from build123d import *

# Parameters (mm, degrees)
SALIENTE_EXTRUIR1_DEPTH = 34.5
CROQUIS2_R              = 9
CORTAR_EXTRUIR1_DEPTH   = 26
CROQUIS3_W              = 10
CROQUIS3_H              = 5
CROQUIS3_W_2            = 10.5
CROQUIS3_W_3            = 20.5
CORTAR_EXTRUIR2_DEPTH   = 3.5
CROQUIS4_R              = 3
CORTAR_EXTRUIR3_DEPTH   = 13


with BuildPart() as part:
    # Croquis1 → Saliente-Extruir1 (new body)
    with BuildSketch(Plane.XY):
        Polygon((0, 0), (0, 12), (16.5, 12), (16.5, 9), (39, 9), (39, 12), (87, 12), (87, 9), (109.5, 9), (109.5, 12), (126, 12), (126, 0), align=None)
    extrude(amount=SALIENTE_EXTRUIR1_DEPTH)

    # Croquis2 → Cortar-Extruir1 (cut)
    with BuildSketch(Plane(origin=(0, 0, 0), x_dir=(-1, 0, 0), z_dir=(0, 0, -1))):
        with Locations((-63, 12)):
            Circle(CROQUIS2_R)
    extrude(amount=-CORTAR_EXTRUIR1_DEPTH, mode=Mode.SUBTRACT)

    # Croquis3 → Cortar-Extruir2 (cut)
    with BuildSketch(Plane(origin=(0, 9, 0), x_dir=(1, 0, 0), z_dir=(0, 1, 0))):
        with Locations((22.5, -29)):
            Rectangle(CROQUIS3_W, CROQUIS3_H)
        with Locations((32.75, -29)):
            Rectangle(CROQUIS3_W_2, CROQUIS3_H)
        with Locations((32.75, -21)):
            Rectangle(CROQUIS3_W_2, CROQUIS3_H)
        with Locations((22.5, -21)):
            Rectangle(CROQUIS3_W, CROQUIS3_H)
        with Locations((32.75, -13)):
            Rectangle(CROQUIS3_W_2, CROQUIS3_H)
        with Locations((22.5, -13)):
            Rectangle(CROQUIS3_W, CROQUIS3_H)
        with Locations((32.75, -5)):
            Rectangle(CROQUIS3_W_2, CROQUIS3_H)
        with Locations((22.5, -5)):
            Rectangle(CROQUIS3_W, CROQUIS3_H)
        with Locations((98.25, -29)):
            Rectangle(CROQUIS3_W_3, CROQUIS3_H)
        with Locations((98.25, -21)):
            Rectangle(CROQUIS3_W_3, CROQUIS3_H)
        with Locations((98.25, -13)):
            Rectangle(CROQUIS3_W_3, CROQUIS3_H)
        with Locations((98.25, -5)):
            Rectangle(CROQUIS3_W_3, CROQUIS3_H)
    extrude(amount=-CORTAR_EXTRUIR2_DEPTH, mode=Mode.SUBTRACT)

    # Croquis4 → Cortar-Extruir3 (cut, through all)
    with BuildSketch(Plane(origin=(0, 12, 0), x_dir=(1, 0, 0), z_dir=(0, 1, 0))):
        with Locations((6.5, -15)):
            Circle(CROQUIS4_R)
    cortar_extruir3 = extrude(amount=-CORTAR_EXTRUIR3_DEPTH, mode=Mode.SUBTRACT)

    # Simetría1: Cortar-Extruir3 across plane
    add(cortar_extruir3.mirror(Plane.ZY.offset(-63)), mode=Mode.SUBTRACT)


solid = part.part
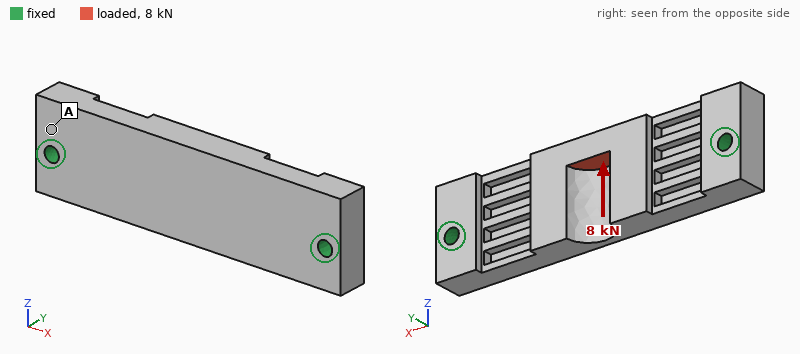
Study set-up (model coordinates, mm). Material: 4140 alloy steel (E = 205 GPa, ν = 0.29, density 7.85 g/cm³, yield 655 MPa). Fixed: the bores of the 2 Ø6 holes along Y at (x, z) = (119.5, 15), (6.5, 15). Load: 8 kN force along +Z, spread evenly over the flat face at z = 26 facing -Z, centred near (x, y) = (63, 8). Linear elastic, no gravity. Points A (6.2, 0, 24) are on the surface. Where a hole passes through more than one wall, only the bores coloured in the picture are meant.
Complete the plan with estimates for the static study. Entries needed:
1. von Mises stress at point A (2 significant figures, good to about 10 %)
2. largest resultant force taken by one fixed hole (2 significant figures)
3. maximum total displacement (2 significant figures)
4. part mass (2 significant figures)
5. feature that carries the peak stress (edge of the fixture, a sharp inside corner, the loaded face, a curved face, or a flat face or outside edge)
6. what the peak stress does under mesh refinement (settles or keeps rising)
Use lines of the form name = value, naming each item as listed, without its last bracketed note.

von Mises stress at point A = 43 MPa
largest resultant force taken by one fixed hole = 5.0 kN
maximum total displacement = 84 µm
part mass = 320 g
feature that carries the peak stress = edge of the fixture
what the peak stress does under mesh refinement = keeps rising
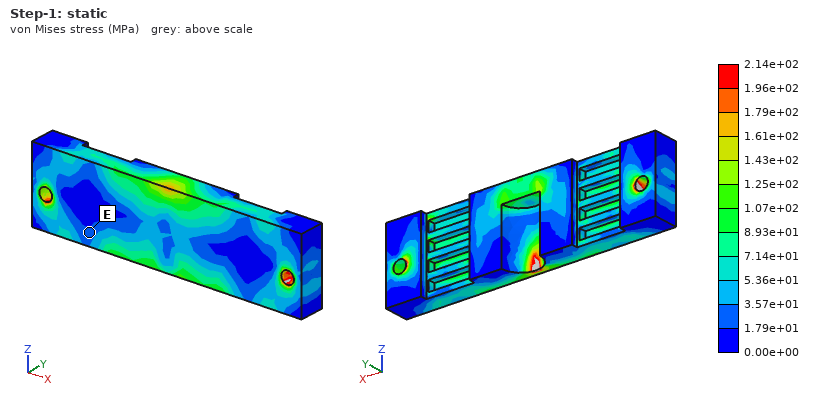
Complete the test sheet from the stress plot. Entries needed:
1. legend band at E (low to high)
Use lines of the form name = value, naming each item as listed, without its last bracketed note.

legend band at E = 1.79e+01 to 3.57e+01 MPa
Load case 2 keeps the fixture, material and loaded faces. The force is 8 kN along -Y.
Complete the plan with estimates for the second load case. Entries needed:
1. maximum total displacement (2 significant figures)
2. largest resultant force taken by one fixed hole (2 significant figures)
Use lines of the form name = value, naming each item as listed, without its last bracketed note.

maximum total displacement = 0.21 mm
largest resultant force taken by one fixed hole = 4.8 kN
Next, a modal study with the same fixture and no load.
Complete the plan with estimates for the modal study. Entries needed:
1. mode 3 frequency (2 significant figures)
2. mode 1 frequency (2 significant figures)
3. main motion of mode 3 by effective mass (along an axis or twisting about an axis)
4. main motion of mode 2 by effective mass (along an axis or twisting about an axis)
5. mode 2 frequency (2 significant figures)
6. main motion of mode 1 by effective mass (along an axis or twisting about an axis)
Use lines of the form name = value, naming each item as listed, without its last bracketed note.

mode 3 frequency = 6600 Hz
mode 1 frequency = 3400 Hz
main motion of mode 3 by effective mass = along Z
main motion of mode 2 by effective mass = along Z
mode 2 frequency = 5400 Hz
main motion of mode 1 by effective mass = along Y
